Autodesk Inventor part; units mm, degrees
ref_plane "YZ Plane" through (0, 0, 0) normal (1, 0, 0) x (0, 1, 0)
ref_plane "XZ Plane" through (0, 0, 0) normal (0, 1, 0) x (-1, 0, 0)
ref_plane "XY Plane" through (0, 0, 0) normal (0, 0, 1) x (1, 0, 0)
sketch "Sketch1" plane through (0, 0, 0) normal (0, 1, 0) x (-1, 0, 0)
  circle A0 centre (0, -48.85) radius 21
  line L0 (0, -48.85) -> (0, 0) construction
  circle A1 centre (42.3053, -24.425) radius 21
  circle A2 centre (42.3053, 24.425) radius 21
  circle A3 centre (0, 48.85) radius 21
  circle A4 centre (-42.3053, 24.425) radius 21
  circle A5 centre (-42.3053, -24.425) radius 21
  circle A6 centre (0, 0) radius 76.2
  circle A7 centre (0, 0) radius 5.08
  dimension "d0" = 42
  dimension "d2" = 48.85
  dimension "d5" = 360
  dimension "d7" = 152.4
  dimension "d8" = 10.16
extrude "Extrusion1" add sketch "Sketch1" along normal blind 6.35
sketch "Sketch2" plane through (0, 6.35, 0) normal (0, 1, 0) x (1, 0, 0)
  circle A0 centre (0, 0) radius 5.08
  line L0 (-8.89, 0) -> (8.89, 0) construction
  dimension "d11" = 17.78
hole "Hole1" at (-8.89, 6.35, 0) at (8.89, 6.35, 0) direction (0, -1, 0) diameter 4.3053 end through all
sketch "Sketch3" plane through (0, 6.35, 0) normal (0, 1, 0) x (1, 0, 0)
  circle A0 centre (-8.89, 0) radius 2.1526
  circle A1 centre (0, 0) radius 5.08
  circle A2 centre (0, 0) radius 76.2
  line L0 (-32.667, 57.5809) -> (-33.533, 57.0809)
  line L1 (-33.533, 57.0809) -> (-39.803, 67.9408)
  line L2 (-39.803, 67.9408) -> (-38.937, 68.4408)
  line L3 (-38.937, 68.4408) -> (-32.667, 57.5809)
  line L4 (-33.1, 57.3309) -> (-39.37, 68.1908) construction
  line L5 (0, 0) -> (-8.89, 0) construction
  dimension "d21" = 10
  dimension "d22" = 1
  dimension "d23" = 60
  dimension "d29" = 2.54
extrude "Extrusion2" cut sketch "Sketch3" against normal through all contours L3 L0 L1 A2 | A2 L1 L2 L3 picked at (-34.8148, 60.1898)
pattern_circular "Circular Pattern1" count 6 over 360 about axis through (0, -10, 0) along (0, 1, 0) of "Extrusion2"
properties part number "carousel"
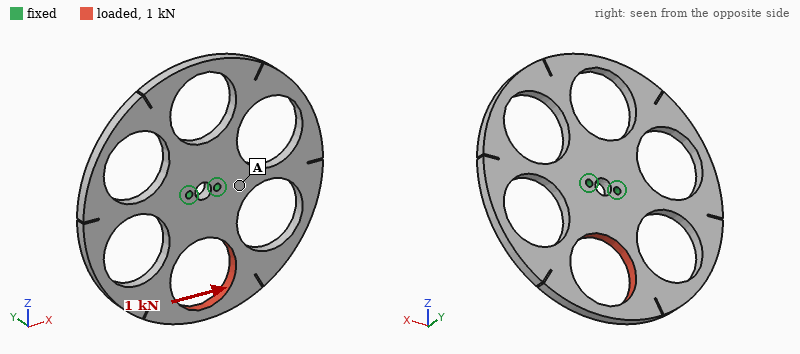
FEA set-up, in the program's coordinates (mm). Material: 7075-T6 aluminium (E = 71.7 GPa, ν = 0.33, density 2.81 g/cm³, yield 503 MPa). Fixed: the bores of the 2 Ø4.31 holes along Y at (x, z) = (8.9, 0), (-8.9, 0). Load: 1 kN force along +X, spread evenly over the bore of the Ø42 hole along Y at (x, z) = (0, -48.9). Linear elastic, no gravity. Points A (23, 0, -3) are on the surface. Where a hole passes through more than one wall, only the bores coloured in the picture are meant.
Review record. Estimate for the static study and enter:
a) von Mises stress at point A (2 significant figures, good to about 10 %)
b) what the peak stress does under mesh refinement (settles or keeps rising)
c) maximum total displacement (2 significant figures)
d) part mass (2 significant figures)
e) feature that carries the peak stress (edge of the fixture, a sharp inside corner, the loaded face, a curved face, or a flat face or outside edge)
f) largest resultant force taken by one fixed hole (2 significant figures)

5.1 MPa
keeps rising
74 µm
170 g
edge of the fixture
2.3 kN
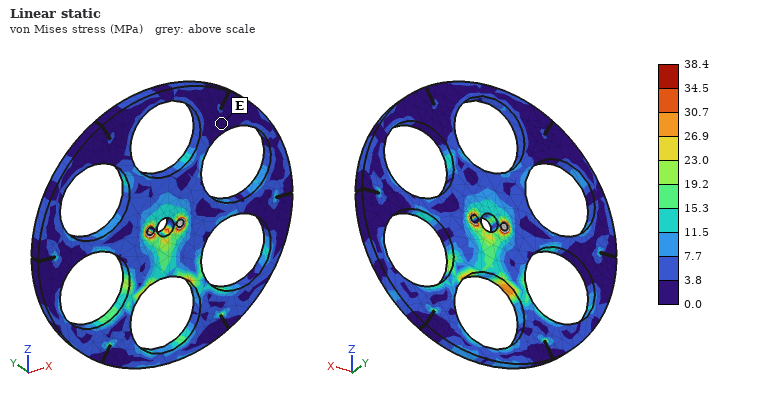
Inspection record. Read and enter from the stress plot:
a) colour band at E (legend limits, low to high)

0.0 to 3.8 MPa
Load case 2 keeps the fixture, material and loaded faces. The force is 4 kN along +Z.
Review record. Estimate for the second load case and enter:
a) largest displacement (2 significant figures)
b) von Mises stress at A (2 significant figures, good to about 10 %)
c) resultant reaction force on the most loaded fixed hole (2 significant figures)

67 µm
7.1 MPa
2.0 kN
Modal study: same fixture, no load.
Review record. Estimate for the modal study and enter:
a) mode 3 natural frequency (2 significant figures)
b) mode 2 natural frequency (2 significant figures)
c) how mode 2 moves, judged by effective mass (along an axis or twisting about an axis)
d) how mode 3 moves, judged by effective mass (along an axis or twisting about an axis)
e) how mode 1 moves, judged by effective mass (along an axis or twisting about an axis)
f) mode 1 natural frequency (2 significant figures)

850 Hz
800 Hz
twisting about Z
along Y
twisting about X
690 Hz
